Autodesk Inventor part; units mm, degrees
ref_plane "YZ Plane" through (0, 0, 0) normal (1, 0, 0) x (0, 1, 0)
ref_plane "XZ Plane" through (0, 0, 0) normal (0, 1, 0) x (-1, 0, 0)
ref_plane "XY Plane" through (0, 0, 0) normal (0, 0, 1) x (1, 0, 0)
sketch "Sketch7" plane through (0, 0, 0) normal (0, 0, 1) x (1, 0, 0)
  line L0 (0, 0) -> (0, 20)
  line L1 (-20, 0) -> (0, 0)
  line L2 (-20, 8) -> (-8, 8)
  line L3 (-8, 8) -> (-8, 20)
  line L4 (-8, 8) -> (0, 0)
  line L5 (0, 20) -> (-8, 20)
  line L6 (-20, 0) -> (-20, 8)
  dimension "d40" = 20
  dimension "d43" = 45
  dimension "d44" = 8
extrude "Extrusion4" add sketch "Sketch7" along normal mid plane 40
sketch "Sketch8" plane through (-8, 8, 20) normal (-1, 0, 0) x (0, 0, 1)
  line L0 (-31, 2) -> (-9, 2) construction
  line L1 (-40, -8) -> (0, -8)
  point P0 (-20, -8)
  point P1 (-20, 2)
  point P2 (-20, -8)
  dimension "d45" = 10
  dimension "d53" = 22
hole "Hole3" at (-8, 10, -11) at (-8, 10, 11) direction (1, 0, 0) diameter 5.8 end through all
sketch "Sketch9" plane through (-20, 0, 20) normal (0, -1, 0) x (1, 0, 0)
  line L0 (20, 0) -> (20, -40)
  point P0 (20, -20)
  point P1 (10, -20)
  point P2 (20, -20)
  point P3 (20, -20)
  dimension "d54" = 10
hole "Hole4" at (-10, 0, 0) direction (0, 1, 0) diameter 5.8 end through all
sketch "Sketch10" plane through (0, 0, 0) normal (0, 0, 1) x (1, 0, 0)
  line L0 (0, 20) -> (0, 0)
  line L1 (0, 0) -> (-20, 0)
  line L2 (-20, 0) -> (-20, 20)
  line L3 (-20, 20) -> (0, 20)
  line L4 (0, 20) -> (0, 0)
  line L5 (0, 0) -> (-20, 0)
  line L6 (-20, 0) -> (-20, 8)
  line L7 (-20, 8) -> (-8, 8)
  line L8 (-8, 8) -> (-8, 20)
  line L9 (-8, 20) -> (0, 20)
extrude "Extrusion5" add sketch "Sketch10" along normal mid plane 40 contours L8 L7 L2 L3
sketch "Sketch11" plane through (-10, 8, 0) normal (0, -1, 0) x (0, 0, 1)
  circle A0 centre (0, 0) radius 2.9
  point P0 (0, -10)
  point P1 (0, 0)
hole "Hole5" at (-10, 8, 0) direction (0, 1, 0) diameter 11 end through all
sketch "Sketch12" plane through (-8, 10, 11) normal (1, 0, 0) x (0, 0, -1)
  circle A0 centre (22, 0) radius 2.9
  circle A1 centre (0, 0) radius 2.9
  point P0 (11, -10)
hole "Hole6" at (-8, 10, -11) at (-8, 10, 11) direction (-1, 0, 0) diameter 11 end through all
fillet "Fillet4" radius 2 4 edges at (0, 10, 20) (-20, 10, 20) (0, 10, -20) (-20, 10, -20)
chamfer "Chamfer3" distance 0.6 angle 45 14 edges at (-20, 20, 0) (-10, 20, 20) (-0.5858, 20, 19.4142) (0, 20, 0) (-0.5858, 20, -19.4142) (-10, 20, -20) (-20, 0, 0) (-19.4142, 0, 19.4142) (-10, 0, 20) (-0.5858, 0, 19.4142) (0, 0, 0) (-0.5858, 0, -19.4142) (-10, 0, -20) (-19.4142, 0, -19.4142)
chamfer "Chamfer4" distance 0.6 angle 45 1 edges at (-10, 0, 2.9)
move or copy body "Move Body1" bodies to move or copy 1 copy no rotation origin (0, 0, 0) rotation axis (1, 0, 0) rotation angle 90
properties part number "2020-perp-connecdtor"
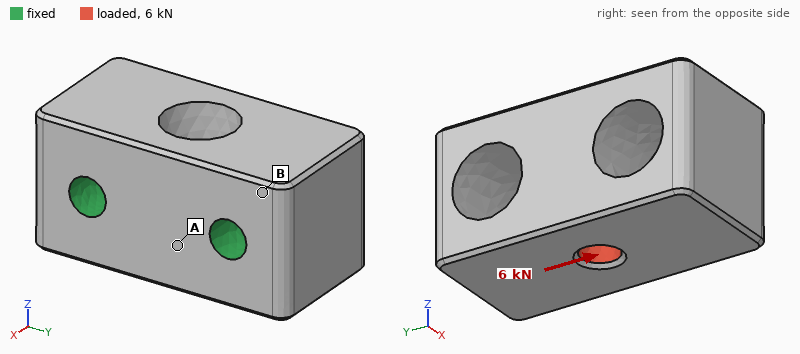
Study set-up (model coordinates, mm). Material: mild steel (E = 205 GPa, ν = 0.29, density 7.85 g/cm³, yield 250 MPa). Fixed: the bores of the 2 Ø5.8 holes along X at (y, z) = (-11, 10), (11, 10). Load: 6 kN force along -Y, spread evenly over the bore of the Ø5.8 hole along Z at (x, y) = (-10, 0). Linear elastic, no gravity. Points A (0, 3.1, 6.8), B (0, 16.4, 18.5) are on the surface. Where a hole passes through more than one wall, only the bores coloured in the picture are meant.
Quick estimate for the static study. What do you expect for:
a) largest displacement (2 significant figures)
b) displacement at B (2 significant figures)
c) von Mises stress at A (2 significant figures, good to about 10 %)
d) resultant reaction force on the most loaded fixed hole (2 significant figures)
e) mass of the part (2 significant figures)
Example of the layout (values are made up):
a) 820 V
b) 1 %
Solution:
a) 4.5 µm
b) 0.91 µm
c) 19 MPa
d) 3.4 kN
e) 93 g
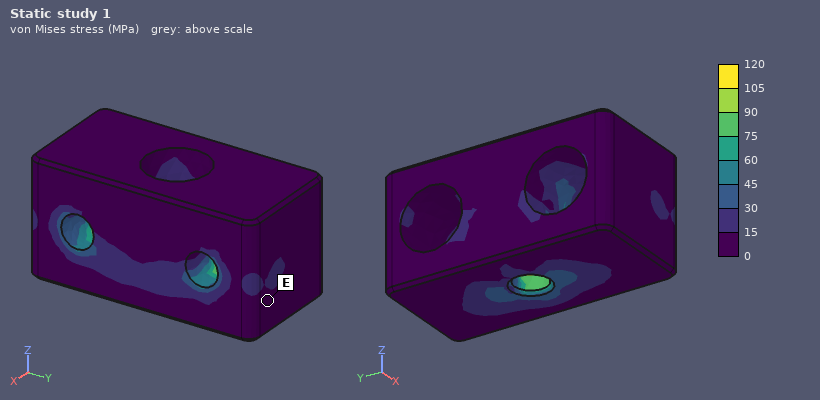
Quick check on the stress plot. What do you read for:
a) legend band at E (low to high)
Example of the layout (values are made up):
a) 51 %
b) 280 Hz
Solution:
a) 0 to 15 MPa
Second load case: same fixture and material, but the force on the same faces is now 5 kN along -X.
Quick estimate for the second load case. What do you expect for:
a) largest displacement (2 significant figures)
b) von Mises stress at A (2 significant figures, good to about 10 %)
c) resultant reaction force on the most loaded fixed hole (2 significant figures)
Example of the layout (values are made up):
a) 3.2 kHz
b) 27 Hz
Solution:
a) 5.8 µm
b) 20 MPa
c) 2.5 kN
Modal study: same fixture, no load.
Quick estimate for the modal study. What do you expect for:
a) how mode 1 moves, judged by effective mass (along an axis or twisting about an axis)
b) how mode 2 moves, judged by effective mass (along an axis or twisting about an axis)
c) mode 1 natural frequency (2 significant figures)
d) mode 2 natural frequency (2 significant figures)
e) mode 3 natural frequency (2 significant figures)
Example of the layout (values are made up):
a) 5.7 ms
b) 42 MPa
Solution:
a) along Z
b) along Y
c) 17 kHz
d) 24 kHz
e) 27 kHz
